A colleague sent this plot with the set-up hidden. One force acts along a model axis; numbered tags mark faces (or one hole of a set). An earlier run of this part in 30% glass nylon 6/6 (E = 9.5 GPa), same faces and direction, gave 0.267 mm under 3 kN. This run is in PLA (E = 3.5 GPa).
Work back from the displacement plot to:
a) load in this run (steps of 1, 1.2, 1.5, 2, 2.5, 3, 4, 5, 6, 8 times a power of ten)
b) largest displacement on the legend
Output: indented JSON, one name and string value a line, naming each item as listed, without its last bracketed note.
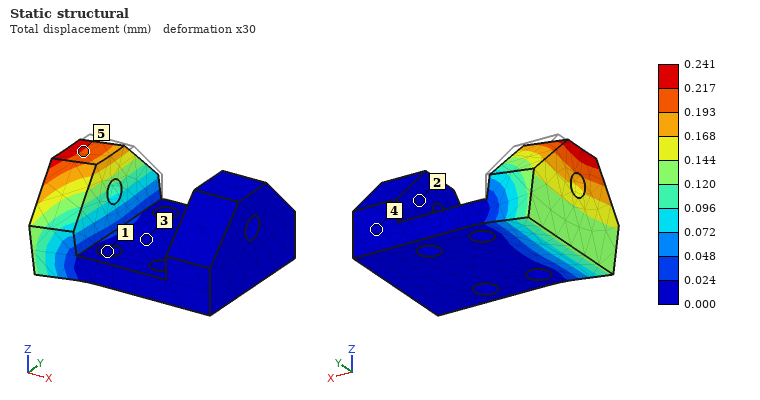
{
  "load in this run": "1 kN",
  "largest displacement on the legend": "0.241 mm"
}
